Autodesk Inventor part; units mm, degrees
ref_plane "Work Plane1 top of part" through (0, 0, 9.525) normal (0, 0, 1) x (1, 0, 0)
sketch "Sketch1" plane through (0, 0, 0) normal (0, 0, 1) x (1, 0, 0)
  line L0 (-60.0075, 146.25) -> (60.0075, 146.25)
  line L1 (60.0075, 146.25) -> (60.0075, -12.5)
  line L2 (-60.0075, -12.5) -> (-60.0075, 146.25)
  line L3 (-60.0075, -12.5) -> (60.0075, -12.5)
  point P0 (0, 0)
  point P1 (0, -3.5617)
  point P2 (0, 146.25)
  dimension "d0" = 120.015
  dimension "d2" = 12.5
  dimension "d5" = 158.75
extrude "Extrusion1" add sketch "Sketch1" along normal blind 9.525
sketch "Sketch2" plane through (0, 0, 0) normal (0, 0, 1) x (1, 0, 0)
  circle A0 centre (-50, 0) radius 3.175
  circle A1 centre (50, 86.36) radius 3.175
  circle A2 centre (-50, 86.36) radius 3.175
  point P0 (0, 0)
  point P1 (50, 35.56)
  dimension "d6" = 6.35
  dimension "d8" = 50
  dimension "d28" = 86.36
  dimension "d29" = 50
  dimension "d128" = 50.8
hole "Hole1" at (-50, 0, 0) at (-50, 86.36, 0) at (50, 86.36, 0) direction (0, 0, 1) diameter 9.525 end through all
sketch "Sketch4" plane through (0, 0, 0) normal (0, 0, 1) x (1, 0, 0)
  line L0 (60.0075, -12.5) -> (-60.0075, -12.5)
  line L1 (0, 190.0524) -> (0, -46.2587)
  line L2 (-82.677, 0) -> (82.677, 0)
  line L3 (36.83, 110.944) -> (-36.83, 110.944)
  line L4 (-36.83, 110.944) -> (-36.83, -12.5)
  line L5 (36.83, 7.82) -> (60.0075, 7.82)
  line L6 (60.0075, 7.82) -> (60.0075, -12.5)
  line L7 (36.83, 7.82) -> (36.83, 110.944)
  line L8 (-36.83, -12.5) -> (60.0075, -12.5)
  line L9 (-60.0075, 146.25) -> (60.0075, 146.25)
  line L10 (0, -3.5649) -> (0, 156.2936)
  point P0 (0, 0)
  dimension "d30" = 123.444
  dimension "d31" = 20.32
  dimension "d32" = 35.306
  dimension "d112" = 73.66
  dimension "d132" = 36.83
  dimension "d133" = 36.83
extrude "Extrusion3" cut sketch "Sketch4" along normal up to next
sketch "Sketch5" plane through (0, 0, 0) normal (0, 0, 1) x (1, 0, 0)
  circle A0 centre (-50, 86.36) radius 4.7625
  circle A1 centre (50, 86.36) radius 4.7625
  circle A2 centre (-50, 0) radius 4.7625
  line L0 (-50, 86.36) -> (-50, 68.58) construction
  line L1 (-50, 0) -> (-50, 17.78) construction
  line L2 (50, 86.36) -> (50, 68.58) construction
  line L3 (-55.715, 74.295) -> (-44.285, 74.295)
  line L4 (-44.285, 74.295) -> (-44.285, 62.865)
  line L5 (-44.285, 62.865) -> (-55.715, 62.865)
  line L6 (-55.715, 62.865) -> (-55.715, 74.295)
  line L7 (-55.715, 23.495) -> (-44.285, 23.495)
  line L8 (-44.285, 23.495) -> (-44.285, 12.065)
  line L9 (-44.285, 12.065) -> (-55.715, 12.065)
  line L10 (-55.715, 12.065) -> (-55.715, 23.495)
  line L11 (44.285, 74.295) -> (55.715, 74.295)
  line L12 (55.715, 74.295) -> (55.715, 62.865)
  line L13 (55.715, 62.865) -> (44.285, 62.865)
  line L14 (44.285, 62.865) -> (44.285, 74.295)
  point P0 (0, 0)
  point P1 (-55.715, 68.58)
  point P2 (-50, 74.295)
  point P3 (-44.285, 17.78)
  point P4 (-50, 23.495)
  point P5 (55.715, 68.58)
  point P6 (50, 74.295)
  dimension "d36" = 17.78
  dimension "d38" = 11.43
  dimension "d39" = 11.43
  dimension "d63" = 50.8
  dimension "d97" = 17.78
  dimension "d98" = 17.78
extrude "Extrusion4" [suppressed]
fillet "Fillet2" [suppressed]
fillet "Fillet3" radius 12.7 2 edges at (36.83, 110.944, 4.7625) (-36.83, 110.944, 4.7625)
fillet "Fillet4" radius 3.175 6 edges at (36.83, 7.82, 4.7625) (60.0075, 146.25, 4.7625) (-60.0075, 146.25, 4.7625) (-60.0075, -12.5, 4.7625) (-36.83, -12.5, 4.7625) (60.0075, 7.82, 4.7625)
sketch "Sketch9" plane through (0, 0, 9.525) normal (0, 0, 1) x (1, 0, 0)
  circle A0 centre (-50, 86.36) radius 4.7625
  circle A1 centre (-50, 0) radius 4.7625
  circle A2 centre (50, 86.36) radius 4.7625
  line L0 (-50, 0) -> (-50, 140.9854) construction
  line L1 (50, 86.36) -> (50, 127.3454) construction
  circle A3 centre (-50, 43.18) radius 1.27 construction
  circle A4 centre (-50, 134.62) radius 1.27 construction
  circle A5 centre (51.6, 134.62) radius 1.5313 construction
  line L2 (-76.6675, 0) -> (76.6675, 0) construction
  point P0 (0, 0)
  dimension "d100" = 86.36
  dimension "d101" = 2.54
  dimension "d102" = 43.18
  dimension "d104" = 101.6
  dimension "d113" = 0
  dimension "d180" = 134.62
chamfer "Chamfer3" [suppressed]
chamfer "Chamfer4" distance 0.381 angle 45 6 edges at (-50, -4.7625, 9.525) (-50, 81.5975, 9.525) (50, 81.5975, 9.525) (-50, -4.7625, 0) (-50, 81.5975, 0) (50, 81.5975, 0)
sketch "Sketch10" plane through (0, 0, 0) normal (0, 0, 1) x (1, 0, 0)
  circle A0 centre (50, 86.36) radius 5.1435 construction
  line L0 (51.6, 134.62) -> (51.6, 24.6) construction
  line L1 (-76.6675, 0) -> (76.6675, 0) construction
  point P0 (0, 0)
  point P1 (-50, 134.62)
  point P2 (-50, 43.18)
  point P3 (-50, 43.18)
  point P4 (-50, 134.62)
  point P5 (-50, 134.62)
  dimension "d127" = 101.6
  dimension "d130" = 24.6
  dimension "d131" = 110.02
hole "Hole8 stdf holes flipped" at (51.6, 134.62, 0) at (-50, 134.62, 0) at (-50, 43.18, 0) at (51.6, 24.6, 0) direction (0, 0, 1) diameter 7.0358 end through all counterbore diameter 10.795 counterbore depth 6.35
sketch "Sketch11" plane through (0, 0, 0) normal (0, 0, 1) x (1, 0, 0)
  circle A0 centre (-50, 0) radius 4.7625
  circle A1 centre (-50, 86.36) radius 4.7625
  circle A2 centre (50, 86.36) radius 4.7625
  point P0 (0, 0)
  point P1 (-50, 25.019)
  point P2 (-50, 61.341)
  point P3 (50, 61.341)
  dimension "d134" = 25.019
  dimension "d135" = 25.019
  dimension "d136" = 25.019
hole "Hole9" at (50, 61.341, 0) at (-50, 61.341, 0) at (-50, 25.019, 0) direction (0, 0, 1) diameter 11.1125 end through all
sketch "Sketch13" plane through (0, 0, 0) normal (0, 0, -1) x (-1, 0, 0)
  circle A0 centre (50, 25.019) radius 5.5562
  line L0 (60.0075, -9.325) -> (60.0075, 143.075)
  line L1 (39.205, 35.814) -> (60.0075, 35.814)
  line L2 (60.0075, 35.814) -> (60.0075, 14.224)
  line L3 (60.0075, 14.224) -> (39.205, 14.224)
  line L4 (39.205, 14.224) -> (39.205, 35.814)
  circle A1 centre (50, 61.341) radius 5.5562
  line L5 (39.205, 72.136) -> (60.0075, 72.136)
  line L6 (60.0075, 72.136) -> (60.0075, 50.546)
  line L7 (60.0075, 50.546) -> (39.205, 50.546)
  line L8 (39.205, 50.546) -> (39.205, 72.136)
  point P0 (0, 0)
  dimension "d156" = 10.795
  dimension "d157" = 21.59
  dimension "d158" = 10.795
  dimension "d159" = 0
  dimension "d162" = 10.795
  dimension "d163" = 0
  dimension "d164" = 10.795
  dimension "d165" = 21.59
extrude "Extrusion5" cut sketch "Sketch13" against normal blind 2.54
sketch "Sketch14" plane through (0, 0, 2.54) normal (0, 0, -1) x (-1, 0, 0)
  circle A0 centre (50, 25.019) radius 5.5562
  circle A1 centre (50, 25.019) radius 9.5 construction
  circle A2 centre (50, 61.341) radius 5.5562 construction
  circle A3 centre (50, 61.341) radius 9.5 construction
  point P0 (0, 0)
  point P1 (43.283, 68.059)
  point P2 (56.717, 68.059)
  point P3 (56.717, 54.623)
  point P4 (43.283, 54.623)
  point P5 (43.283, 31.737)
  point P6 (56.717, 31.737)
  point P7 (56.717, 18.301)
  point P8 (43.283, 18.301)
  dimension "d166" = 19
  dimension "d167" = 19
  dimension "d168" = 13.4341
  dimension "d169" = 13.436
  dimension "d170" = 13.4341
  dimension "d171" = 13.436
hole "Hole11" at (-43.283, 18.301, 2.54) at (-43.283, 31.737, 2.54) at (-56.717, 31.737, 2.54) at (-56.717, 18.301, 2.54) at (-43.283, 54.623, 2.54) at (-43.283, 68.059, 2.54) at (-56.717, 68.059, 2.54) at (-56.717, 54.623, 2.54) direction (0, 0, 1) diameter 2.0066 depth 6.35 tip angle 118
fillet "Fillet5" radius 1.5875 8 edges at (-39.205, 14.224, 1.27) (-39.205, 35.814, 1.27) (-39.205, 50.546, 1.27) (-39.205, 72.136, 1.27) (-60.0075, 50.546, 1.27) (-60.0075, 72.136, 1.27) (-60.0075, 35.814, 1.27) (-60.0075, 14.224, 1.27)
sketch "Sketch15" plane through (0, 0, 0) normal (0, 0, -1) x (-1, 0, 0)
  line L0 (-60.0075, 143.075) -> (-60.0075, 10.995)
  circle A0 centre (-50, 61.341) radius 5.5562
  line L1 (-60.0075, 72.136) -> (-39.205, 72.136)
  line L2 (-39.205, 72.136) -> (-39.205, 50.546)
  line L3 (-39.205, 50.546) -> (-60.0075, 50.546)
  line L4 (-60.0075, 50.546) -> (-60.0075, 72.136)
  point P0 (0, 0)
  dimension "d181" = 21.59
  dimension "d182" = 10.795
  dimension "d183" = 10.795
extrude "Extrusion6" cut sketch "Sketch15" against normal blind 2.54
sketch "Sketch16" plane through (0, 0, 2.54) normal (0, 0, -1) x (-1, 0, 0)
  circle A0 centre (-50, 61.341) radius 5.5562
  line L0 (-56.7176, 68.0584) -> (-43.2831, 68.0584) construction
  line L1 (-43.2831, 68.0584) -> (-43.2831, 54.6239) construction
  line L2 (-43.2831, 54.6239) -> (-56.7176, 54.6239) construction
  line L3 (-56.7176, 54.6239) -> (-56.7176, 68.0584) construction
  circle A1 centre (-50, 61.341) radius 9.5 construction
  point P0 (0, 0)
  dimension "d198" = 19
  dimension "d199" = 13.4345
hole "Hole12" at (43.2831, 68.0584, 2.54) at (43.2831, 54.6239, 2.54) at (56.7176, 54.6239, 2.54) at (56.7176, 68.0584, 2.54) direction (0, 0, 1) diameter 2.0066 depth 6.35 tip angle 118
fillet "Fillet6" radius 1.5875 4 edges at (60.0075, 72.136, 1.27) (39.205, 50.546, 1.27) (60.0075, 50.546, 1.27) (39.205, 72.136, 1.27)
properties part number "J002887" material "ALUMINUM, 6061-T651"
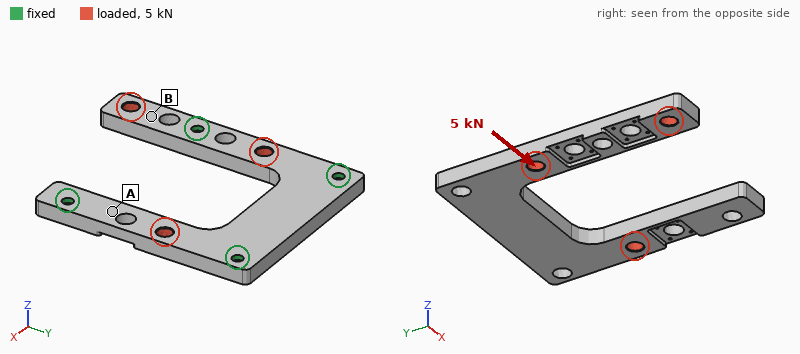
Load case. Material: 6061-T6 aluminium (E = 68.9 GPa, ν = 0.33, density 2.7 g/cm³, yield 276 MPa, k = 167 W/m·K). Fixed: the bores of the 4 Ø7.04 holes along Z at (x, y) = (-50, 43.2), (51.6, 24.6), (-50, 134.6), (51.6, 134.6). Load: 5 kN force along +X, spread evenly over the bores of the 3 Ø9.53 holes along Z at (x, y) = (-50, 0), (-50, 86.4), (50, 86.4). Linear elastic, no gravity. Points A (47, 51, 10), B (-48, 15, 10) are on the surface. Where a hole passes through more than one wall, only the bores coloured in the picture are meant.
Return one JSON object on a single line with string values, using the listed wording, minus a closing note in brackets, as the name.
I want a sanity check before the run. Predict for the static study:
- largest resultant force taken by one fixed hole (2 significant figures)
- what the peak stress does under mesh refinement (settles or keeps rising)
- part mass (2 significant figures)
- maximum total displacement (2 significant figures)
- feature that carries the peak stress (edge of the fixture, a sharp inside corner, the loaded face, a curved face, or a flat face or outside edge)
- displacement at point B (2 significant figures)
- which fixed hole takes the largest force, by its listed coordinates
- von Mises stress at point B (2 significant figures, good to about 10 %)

{"largest resultant force taken by one fixed hole": "2.9 kN", "what the peak stress does under mesh refinement": "keeps rising", "part mass": "220 g", "maximum total displacement": "0.30 mm", "feature that carries the peak stress": "edge of the fixture", "displacement at point B": "0.12 mm", "which fixed hole takes the largest force, by its listed coordinates": "(-50, 43.2)", "von Mises stress at point B": "31 MPa"}
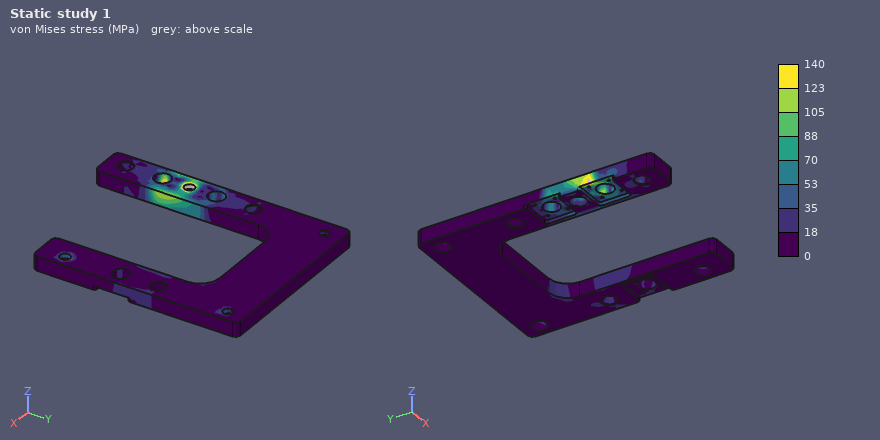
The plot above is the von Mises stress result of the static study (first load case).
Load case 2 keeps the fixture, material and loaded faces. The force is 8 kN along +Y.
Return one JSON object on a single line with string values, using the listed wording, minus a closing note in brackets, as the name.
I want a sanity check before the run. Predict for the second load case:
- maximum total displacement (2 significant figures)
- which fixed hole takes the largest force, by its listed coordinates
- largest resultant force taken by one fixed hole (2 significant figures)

{"maximum total displacement": "0.16 mm", "which fixed hole takes the largest force, by its listed coordinates": "(-50, 43.2)", "largest resultant force taken by one fixed hole": "3.4 kN"}
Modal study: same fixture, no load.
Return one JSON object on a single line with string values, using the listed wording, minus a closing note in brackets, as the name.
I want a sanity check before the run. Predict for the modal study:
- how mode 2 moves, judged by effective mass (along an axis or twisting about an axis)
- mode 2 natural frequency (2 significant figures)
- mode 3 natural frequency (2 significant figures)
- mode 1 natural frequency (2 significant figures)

{"how mode 2 moves, judged by effective mass": "along Z", "mode 2 natural frequency": "2800 Hz", "mode 3 natural frequency": "3400 Hz", "mode 1 natural frequency": "1500 Hz"}
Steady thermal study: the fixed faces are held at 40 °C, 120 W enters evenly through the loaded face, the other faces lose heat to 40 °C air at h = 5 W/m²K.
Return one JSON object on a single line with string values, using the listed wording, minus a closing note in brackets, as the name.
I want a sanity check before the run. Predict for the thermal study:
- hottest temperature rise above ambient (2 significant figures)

{"hottest temperature rise above ambient": "85 K"}
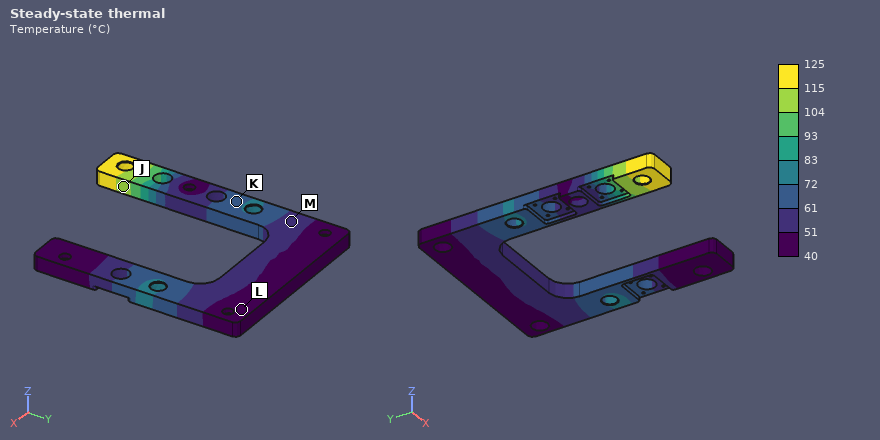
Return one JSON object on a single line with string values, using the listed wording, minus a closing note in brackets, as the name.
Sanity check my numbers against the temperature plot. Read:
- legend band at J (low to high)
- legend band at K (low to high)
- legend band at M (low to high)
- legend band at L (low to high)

{"legend band at J": "104 to 115 °C", "legend band at K": "61 to 72 °C", "legend band at M": "51 to 61 °C", "legend band at L": "40 to 51 °C"}
